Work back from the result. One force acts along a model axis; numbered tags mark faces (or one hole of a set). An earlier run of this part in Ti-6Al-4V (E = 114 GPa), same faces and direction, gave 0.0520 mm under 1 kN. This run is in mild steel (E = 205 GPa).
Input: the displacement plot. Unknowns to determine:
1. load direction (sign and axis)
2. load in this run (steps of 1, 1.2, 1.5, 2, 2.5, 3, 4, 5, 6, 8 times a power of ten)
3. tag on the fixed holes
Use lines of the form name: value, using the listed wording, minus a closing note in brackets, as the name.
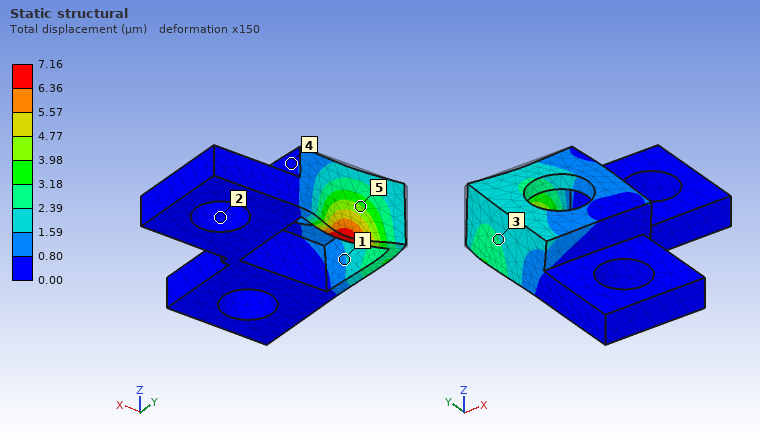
load direction: -Y
load in this run: 250 N
tag on the fixed holes: 2
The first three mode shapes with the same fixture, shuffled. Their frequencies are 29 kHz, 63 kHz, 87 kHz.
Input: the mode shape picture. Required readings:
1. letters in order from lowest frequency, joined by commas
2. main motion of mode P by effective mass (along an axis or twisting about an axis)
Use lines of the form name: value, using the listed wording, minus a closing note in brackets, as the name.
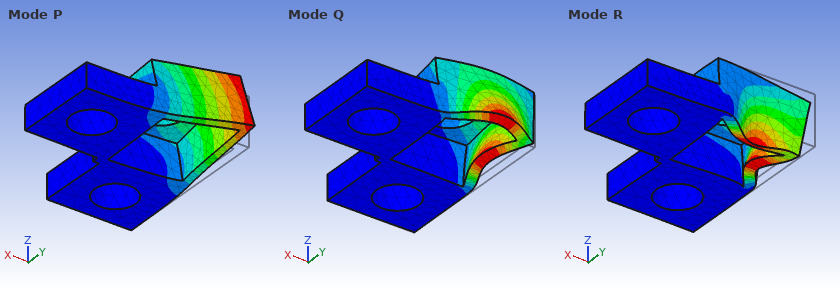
letters in order from lowest frequency, joined by commas: P, Q, R
main motion of mode P by effective mass: along Z
